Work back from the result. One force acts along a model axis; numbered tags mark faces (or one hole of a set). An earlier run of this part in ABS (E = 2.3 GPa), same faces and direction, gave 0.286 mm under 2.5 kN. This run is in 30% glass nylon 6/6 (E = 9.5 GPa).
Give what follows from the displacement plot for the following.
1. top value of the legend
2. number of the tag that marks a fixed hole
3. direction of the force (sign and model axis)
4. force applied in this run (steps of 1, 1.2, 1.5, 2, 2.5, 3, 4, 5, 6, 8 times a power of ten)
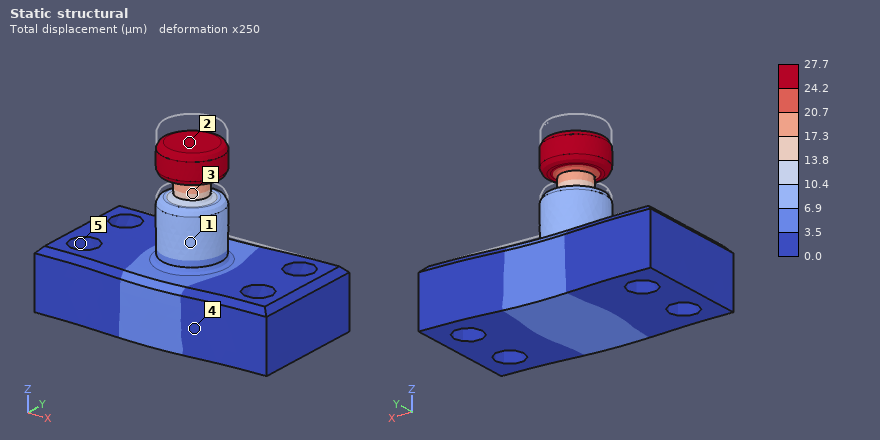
27.7 µm
5
-Z
1 kN
